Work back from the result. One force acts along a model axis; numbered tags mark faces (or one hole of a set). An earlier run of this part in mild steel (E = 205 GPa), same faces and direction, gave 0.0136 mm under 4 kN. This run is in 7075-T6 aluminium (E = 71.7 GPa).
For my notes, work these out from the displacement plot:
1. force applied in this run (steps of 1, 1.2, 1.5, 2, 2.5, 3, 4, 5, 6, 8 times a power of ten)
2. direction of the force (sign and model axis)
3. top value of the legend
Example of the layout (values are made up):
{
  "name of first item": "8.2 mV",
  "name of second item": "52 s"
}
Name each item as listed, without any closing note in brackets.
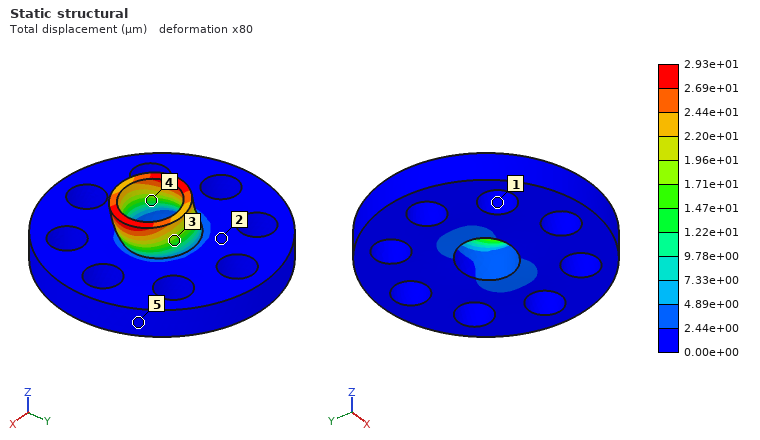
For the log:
{
  "force applied in this run": "3 kN",
  "direction of the force": "+X",
  "top value of the legend": "2.93e+01 µm"
}
